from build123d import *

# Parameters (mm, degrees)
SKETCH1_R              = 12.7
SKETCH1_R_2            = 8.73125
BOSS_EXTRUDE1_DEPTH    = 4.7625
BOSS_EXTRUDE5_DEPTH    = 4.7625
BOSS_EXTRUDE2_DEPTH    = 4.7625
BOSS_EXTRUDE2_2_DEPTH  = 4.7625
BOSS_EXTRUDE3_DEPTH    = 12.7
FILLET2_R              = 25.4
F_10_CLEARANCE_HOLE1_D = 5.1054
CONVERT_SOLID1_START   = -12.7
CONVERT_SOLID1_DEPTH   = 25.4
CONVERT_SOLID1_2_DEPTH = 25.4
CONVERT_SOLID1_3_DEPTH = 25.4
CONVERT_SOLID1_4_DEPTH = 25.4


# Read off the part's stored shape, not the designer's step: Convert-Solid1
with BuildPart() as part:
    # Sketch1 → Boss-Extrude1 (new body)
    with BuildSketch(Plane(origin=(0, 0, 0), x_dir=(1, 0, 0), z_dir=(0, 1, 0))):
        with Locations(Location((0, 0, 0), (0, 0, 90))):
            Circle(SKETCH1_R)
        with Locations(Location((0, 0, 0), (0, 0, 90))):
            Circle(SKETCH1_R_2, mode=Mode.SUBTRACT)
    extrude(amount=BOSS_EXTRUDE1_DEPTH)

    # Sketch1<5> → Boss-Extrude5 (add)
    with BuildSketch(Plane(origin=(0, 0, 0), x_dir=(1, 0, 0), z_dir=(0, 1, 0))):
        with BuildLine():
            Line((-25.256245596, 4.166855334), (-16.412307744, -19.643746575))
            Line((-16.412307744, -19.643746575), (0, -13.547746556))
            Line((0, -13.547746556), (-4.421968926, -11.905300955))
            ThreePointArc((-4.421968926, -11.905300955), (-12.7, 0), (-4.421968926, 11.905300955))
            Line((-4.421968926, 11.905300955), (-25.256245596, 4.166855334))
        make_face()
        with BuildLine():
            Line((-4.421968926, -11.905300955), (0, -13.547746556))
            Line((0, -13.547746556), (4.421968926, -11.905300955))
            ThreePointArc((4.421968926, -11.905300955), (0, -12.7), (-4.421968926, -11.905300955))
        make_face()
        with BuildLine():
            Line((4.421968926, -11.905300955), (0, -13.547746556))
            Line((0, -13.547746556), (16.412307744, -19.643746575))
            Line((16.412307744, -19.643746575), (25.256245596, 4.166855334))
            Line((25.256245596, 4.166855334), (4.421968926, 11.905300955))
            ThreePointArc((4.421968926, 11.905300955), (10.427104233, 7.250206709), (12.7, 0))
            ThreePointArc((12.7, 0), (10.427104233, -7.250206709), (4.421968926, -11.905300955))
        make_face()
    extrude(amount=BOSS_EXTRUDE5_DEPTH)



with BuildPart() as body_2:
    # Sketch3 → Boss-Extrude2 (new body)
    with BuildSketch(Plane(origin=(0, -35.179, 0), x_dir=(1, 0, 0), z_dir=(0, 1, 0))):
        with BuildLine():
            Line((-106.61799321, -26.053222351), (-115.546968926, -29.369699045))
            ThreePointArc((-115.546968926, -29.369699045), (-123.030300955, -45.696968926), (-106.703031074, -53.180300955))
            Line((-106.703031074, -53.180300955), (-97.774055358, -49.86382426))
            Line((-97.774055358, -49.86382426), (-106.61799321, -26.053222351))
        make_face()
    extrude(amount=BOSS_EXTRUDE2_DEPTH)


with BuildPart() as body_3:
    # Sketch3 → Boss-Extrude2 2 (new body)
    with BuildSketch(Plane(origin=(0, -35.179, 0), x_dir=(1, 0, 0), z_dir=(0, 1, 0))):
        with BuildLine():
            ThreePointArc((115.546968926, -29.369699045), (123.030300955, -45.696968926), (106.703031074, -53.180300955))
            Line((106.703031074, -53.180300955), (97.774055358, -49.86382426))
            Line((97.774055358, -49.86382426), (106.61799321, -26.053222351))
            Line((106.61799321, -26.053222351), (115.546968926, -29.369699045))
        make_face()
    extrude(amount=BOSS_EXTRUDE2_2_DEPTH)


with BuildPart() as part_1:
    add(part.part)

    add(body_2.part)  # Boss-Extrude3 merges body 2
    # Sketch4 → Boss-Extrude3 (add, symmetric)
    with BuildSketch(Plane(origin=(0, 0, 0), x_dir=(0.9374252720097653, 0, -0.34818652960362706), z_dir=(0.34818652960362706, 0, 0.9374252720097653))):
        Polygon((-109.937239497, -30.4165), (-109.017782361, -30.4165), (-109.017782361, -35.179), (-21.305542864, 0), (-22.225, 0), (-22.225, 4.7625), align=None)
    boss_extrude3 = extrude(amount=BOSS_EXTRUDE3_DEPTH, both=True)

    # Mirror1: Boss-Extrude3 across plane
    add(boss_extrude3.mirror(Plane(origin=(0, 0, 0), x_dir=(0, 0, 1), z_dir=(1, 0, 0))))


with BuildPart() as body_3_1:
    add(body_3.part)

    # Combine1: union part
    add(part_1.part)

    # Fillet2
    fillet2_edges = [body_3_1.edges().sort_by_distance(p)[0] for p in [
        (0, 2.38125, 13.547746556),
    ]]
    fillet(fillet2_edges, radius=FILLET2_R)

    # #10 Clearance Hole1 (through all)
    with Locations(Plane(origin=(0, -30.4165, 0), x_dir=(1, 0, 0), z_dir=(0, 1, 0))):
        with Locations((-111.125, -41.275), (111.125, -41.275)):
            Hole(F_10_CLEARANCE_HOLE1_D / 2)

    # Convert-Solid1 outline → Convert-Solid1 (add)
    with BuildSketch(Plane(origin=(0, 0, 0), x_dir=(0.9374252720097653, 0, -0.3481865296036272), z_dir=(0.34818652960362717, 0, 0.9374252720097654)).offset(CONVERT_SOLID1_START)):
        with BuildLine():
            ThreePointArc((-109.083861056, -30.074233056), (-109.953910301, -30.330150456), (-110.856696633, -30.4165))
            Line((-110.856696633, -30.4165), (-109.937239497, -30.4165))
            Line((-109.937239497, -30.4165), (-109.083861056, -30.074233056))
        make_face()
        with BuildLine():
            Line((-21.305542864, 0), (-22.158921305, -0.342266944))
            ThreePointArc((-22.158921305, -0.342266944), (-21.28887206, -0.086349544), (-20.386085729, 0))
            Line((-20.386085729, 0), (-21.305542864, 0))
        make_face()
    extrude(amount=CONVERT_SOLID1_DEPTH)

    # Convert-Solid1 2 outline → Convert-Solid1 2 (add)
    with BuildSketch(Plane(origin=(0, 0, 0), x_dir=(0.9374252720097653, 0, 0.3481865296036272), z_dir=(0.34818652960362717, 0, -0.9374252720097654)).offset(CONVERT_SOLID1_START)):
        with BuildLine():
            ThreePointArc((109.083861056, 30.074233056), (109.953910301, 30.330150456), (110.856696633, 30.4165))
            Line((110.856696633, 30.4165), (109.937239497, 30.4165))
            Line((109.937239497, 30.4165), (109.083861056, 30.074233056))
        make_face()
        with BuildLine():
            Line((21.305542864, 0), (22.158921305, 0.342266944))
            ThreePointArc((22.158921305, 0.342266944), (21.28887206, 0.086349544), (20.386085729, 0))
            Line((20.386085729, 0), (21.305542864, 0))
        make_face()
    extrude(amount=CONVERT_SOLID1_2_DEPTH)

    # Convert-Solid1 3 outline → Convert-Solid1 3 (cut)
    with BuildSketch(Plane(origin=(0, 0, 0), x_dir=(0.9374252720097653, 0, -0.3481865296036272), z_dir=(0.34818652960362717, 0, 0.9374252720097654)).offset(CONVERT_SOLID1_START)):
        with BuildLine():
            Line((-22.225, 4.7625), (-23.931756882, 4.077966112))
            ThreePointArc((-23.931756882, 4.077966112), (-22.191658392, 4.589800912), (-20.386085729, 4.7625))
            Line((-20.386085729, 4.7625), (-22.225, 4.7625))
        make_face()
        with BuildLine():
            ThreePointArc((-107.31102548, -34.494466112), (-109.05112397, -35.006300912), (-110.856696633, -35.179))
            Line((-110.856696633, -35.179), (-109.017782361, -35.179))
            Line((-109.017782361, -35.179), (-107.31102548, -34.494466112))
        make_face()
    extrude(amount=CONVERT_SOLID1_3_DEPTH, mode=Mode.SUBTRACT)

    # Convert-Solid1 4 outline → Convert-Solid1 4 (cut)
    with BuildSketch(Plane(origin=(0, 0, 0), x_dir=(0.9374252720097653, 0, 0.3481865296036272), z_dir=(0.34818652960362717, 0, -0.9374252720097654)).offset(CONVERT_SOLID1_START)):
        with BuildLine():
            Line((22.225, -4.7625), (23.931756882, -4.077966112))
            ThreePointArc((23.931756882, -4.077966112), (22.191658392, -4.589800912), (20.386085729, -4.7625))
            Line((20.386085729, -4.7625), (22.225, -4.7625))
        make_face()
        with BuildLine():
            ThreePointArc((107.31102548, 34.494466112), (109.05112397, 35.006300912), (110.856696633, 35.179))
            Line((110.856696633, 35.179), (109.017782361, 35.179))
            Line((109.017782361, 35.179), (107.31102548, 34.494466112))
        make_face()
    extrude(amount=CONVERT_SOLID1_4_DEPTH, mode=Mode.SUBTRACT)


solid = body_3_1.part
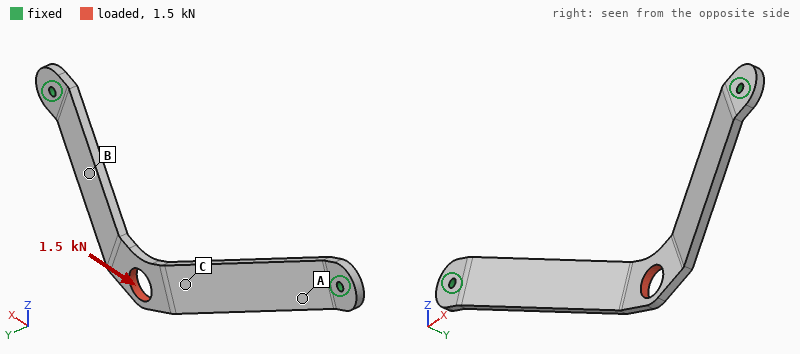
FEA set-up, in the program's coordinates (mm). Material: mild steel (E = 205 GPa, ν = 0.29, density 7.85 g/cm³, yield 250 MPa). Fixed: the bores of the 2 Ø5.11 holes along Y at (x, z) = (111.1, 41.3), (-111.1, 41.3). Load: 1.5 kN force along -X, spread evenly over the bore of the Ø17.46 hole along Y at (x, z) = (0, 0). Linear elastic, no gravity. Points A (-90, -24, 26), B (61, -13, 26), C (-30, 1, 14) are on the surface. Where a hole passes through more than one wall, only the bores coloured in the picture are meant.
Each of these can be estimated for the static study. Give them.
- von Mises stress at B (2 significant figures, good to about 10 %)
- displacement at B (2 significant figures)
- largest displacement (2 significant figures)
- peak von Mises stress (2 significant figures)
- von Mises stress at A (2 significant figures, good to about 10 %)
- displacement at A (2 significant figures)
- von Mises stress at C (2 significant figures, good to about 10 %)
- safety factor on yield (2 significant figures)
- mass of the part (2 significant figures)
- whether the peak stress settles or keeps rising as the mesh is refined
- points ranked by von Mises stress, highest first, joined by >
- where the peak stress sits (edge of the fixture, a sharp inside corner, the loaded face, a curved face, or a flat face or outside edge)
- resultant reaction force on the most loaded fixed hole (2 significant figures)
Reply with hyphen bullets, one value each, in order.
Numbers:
- 6.9 MPa
- 52 µm
- 87 µm
- 68 MPa
- 23 MPa
- 17 µm
- 33 MPa
- 3.7
- 250 g
- settles
- C > A > B
- a curved face
- 830 N
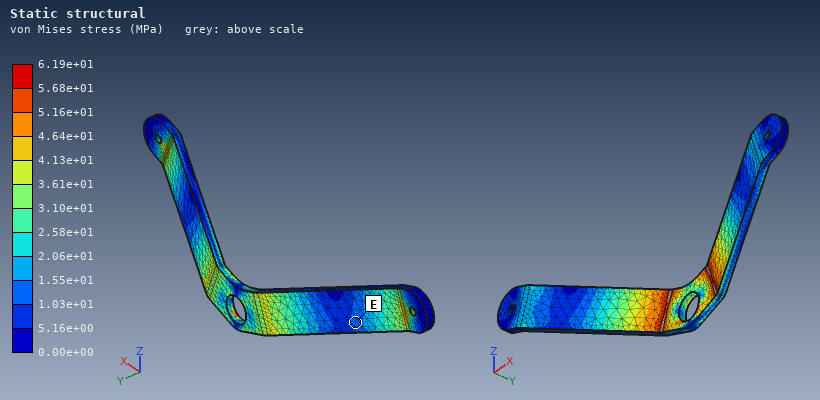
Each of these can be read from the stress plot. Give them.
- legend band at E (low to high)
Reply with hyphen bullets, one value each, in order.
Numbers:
- 1.03e+01 to 1.55e+01 MPa
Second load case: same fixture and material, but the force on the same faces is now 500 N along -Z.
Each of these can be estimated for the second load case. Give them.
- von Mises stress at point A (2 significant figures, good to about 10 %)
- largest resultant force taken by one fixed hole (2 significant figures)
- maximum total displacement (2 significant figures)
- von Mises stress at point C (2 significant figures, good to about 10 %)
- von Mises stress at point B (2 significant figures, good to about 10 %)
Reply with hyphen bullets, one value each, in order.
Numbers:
- 23 MPa
- 250 N
- 0.27 mm
- 21 MPa
- 25 MPa
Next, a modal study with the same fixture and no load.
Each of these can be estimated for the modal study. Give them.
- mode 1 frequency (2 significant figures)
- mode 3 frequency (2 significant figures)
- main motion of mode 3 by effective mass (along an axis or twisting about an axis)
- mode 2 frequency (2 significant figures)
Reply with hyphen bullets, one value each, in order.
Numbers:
- 700 Hz
- 1800 Hz
- along Y
- 1100 Hz
